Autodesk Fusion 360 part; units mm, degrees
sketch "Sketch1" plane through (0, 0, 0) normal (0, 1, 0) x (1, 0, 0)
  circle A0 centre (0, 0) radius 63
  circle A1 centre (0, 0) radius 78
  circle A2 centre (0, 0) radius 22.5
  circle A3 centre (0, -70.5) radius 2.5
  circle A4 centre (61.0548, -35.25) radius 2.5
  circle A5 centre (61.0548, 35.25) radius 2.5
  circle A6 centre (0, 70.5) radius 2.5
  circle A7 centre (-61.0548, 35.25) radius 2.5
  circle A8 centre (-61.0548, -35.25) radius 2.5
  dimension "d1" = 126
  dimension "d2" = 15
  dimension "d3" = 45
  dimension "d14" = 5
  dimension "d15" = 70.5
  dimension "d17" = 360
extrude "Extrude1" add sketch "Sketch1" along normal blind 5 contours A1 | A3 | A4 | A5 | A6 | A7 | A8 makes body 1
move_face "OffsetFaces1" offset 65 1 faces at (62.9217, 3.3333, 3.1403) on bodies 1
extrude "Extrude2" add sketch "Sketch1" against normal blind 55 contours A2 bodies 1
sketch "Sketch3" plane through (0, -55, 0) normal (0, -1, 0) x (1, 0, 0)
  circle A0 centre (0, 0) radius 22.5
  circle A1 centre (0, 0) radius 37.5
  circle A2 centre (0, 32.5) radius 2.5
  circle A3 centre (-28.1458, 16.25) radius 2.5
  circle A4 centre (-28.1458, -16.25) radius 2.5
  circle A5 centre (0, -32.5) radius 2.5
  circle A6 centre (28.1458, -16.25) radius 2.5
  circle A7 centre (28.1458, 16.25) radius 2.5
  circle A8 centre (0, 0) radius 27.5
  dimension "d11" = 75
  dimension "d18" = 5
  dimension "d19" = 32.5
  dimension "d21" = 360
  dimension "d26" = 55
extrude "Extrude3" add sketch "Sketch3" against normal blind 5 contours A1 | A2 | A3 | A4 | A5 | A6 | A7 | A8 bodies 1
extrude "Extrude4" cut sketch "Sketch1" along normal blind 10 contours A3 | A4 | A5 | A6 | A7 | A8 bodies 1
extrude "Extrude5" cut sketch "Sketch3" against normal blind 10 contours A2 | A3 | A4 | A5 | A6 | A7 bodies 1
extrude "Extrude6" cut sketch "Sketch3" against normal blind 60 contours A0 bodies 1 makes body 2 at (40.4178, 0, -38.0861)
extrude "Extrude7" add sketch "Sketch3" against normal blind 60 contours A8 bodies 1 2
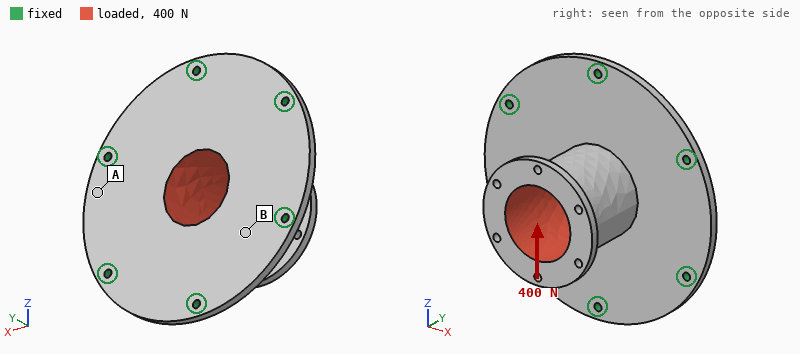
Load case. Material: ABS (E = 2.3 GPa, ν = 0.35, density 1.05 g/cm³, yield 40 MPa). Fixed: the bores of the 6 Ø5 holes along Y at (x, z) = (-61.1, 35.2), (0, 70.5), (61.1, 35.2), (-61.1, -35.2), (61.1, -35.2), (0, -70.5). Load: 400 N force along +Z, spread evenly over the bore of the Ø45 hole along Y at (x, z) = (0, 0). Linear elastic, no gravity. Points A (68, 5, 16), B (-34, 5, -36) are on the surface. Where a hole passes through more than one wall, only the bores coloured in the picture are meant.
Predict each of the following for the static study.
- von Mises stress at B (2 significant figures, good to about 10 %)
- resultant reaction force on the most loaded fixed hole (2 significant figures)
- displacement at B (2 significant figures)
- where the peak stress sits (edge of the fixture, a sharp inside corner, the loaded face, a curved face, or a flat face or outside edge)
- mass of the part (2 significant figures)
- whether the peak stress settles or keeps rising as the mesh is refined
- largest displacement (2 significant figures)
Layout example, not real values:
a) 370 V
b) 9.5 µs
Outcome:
a) 1.9 MPa
b) 120 N
c) 0.15 mm
d) edge of the fixture
e) 150 g
f) keeps rising
g) 0.86 mm
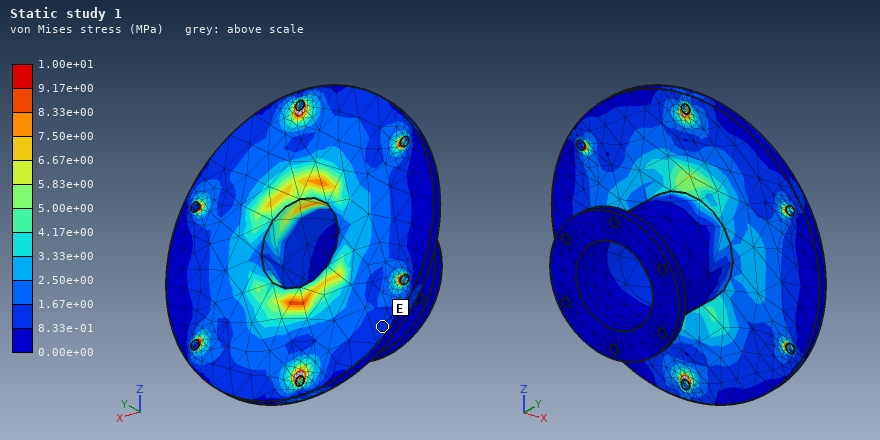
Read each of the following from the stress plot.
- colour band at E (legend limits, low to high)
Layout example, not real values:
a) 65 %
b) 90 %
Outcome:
a) 8.33e-01 to 1.67e+00 MPa
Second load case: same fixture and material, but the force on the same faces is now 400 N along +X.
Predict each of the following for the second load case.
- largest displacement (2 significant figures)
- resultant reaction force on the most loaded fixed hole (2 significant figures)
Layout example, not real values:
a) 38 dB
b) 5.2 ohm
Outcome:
a) 0.87 mm
b) 110 N
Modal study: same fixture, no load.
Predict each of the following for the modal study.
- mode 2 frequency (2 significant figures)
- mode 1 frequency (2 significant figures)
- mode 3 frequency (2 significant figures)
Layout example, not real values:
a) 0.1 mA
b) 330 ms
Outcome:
a) 440 Hz
b) 440 Hz
c) 450 Hz
